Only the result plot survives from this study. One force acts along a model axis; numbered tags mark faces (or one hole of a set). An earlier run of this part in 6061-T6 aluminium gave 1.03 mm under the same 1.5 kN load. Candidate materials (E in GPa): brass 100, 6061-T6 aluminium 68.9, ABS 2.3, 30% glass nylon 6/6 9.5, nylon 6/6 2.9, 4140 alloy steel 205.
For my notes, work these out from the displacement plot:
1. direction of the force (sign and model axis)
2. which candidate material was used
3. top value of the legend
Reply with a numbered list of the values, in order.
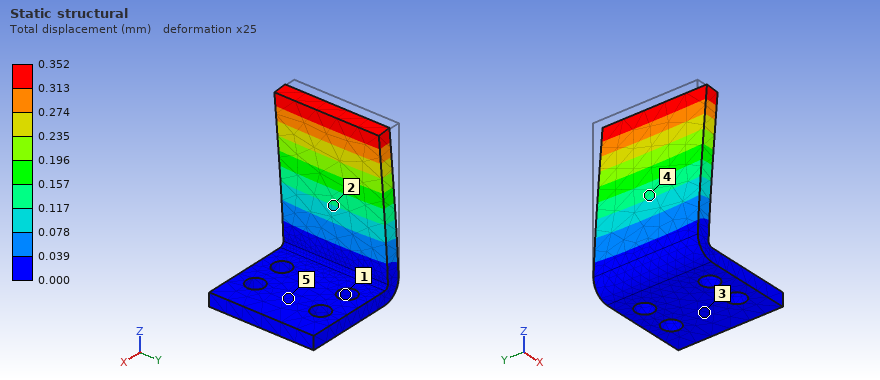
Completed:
1. +X
2. 4140 alloy steel
3. 0.352 mm
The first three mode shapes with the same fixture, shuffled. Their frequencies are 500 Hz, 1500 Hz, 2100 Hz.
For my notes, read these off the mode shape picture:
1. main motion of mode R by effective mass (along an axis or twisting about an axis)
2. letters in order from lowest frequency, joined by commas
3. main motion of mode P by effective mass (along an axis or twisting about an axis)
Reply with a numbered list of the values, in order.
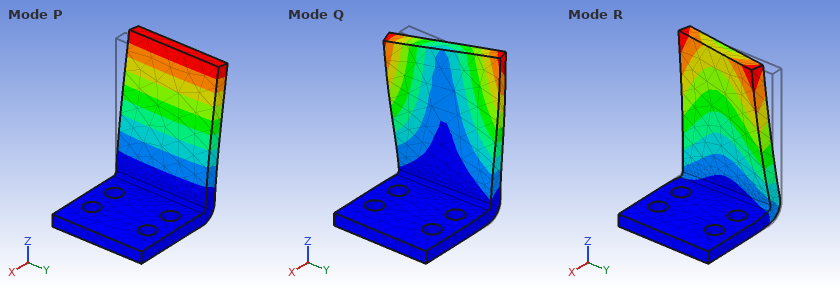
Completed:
1. along Y
2. P, R, Q
3. along X
